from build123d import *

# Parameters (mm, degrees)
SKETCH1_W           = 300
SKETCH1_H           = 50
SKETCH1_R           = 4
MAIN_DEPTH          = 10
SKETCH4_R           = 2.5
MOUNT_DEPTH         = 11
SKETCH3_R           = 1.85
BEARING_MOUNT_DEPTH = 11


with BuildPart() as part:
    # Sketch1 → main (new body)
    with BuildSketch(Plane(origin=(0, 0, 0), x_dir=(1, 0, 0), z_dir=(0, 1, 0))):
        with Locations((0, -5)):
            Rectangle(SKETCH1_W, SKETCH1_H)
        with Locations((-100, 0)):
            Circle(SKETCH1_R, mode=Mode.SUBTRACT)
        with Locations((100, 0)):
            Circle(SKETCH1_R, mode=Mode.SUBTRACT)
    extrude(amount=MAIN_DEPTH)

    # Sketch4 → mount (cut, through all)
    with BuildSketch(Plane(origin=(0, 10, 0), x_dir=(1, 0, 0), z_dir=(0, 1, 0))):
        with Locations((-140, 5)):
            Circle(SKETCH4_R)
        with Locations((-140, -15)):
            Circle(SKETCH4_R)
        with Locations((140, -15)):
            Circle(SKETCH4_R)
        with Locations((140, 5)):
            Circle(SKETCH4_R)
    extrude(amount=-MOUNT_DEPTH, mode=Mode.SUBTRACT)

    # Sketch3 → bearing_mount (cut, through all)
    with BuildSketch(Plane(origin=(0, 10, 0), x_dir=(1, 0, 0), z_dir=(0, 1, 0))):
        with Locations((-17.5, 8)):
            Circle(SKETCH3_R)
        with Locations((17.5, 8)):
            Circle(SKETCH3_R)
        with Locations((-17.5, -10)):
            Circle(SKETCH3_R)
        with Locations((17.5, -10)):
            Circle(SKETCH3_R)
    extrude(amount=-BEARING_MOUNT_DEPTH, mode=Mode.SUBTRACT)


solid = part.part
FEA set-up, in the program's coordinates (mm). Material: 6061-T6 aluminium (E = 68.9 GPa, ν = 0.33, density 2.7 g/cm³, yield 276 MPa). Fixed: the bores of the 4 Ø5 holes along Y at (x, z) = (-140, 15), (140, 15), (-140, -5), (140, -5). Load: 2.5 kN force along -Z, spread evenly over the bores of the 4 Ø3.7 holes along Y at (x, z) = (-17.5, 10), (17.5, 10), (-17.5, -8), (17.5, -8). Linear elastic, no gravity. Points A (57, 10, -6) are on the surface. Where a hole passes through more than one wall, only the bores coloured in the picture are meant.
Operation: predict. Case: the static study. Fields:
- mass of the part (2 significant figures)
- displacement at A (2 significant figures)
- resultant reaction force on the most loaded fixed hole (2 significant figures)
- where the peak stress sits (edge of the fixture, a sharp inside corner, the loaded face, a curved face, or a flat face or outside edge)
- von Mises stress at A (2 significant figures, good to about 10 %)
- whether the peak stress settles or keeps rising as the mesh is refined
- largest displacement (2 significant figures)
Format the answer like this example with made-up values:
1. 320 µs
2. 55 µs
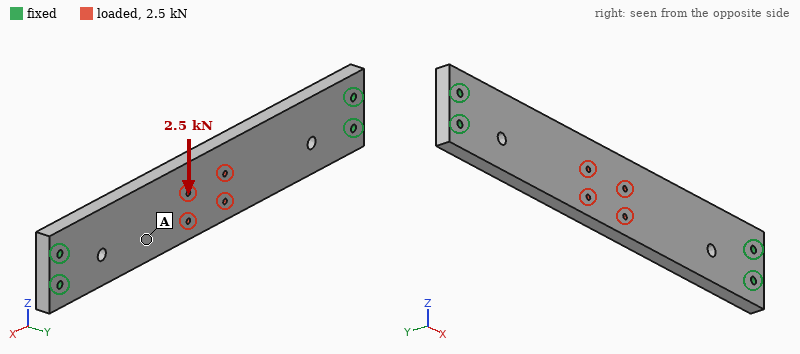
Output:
1. 400 g
2. 48 µm
3. 3.2 kN
4. edge of the fixture
5. 6.1 MPa
6. keeps rising
7. 69 µm
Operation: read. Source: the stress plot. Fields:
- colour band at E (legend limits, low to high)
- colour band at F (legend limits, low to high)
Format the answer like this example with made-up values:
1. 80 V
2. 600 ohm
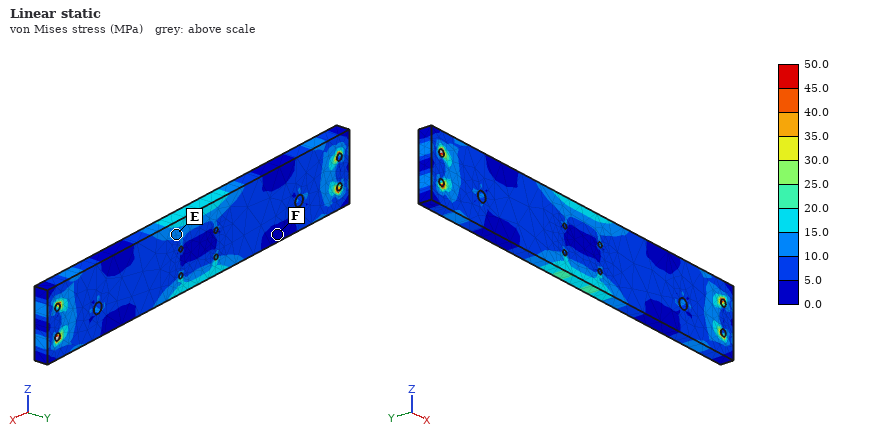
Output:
1. 10.0 to 15.0 MPa
2. 0.0 to 5.0 MPa
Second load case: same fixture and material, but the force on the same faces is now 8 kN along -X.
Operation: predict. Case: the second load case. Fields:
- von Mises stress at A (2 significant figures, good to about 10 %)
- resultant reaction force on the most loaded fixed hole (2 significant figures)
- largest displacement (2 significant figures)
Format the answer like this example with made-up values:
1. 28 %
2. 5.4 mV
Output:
1. 8.8 MPa
2. 2.2 kN
3. 18 µm
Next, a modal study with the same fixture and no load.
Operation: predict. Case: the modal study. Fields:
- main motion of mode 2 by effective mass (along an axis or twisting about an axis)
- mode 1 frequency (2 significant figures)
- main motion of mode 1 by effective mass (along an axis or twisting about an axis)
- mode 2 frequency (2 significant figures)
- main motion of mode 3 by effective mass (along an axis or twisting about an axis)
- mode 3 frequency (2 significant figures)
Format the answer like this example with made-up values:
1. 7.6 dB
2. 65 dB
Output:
1. twisting about Z
2. 650 Hz
3. along Y
4. 1800 Hz
5. twisting about X
6. 2100 Hz
